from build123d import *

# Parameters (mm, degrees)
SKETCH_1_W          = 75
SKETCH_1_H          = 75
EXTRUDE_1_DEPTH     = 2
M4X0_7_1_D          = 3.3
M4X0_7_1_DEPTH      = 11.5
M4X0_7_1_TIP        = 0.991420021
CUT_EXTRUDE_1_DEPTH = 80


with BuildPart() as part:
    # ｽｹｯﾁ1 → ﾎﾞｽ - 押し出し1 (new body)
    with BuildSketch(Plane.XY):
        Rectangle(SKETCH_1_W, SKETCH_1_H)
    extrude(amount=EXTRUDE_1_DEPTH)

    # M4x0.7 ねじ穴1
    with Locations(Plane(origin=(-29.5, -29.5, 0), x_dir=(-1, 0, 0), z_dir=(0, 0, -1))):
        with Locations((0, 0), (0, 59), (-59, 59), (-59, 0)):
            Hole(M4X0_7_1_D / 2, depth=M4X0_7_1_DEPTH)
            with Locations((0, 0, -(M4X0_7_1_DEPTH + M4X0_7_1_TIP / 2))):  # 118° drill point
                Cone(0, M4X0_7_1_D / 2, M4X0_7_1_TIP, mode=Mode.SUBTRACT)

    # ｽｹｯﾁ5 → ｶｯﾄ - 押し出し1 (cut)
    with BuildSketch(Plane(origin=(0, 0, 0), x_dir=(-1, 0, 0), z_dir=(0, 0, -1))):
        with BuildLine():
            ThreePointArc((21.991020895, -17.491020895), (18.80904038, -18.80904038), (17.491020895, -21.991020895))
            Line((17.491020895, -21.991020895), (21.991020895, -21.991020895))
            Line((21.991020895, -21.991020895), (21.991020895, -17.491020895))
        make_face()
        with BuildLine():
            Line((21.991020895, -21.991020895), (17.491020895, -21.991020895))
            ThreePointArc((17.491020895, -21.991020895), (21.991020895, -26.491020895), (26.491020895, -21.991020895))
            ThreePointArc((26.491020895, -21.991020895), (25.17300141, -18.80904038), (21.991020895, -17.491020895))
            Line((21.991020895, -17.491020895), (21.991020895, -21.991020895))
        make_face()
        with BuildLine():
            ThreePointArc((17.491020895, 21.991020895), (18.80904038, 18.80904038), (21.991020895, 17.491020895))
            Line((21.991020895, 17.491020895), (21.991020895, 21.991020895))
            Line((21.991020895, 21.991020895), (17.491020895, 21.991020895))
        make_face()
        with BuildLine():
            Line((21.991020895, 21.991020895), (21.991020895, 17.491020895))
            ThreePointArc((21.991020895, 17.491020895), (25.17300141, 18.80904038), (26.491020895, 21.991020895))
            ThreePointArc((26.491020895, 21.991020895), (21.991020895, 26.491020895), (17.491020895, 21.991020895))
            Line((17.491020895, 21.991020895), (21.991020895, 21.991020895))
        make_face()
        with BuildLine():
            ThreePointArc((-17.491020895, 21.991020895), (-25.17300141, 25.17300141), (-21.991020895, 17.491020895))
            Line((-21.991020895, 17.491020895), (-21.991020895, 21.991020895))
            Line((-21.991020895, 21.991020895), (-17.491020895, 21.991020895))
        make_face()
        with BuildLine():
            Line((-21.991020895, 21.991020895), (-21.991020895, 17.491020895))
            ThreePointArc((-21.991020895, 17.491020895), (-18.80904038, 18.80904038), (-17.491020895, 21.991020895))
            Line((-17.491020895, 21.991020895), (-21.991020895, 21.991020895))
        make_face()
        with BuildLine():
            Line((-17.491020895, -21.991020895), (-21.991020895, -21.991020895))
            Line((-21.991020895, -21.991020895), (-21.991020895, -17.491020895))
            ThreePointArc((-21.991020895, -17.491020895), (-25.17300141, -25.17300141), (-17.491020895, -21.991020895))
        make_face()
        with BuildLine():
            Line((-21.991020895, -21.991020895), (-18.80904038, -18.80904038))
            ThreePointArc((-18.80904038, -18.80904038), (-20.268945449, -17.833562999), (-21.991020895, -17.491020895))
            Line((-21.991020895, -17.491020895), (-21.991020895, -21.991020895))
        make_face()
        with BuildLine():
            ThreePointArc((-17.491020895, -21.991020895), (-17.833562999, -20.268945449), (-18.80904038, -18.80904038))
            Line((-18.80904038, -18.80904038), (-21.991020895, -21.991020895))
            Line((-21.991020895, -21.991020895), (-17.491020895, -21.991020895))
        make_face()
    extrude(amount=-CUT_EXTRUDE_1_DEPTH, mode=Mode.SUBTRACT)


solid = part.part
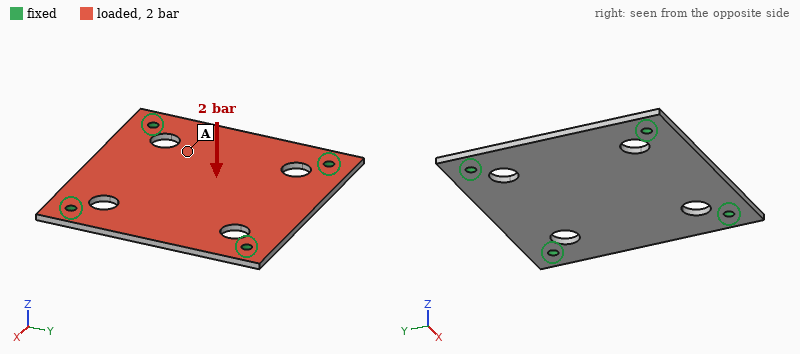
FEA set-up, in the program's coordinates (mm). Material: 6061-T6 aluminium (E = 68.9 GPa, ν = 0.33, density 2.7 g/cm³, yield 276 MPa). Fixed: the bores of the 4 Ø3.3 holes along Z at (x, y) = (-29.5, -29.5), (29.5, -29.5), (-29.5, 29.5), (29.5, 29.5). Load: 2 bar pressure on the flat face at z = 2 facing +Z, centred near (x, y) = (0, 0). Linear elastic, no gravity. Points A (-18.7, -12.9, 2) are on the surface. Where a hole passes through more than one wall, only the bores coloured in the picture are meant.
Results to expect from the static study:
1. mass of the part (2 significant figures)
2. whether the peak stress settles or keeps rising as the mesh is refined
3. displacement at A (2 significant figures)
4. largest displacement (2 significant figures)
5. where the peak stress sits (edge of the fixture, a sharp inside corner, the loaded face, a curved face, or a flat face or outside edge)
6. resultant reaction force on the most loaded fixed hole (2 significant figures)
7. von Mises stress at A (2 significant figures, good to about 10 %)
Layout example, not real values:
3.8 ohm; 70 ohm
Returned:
29 g; keeps rising; 0.22 mm; 0.36 mm; edge of the fixture; 270 N; 33 MPa
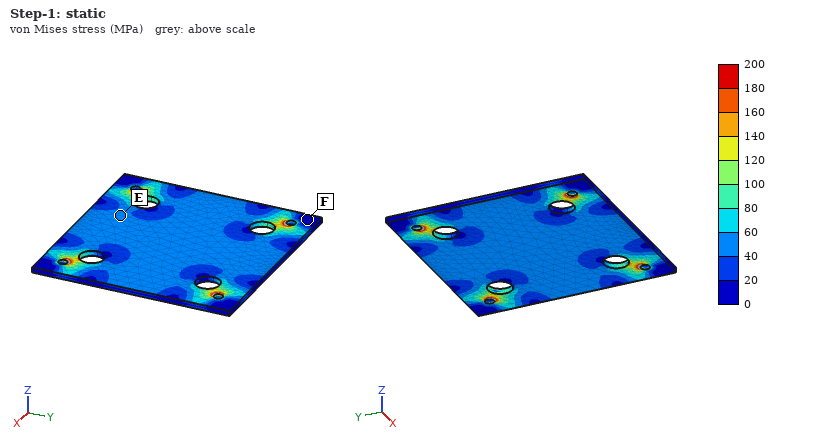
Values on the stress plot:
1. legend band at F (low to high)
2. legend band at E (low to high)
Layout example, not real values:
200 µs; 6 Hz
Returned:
0 to 20 MPa; 40 to 60 MPa
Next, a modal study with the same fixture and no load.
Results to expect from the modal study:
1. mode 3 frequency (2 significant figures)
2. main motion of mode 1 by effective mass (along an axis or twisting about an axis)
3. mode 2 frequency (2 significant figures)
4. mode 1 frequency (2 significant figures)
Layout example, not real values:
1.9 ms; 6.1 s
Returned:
3200 Hz; along Z; 3200 Hz; 2000 Hz
